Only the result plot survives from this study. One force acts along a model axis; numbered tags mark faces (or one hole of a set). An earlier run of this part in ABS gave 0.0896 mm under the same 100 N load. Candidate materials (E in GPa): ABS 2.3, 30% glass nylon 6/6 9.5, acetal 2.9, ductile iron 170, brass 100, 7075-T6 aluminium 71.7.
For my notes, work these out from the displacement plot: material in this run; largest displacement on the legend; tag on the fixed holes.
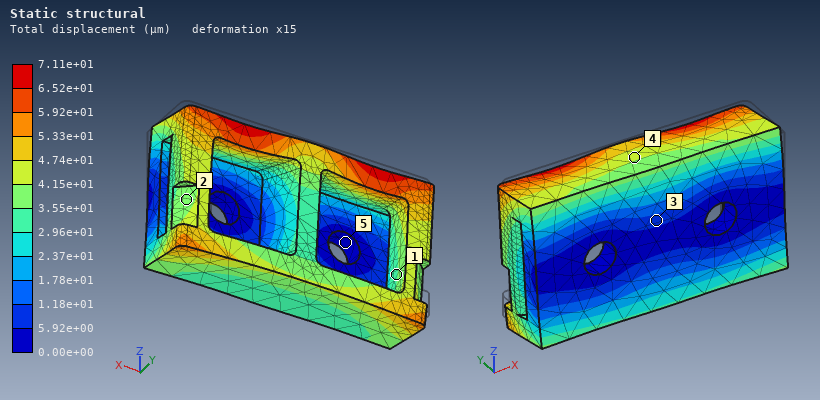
acetal
7.11e+01 µm
5
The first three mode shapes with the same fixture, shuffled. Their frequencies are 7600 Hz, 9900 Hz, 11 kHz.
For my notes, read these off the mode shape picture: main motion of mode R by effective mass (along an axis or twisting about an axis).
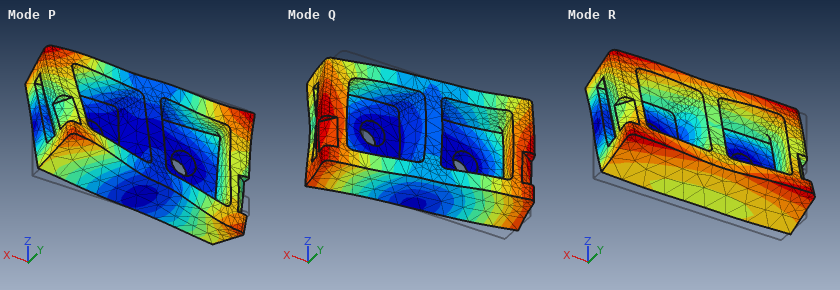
along Z
